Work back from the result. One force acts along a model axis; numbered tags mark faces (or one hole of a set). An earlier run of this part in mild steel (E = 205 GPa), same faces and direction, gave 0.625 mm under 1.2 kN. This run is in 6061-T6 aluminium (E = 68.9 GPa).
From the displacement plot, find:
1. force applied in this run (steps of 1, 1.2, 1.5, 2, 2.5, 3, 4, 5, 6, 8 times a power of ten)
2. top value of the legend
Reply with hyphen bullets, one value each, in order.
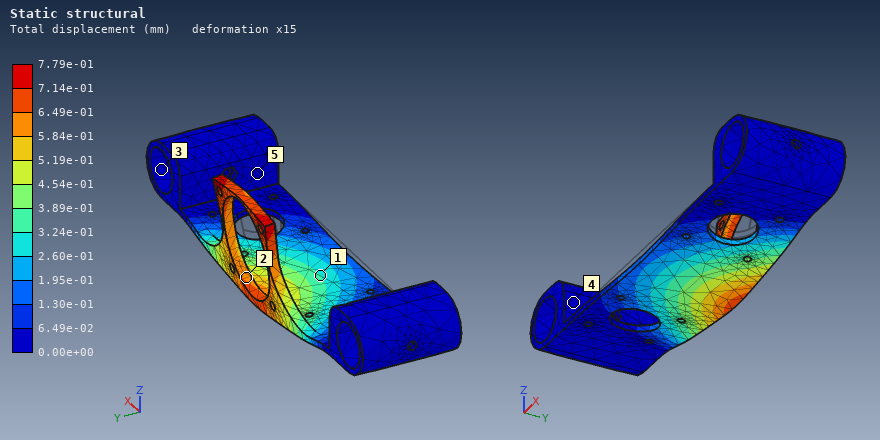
- 500 N
- 7.79e-01 mm
